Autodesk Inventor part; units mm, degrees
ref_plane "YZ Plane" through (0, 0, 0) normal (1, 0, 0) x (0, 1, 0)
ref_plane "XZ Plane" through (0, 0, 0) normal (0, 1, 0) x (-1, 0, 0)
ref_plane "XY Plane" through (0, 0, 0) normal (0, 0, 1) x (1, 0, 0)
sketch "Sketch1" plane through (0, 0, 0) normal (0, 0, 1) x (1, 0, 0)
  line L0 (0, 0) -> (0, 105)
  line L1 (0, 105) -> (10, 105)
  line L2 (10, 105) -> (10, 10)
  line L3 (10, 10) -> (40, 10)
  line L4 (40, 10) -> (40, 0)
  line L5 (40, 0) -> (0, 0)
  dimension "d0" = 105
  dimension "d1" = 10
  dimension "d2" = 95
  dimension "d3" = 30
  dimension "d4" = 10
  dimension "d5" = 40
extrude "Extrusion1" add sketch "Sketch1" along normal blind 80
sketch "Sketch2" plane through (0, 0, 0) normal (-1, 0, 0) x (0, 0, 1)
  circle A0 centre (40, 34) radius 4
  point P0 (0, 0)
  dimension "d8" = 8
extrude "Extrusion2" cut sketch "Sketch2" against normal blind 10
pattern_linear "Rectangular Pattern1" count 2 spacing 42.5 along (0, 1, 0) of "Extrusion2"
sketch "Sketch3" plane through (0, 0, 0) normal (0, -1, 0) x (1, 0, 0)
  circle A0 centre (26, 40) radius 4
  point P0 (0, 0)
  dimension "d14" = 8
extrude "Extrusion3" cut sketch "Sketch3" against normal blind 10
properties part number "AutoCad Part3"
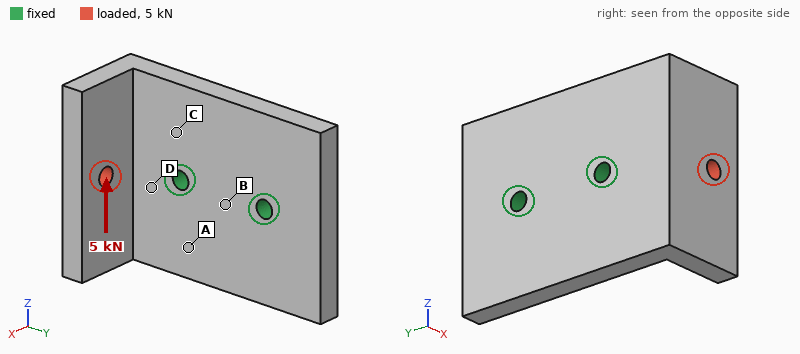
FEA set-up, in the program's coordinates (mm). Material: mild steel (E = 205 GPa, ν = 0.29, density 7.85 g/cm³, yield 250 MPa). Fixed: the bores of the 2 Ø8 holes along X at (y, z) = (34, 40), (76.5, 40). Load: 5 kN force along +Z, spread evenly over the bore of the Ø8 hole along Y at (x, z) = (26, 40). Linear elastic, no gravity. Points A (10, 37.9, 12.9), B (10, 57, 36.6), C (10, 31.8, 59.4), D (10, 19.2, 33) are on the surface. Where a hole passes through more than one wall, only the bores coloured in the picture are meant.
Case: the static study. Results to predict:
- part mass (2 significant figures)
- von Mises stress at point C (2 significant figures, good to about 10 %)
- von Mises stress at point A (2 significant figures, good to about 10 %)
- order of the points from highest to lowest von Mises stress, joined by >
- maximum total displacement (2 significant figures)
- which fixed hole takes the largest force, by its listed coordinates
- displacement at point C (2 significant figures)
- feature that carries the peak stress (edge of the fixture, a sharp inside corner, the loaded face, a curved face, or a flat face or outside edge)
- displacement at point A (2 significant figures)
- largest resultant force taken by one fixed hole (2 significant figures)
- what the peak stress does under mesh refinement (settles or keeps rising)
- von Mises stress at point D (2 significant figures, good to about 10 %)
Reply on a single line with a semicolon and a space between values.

840 g; 42 MPa; 32 MPa; D > C > A > B; 88 µm; (34, 40); 15 µm; edge of the fixture; 19 µm; 7.8 kN; keeps rising; 66 MPa
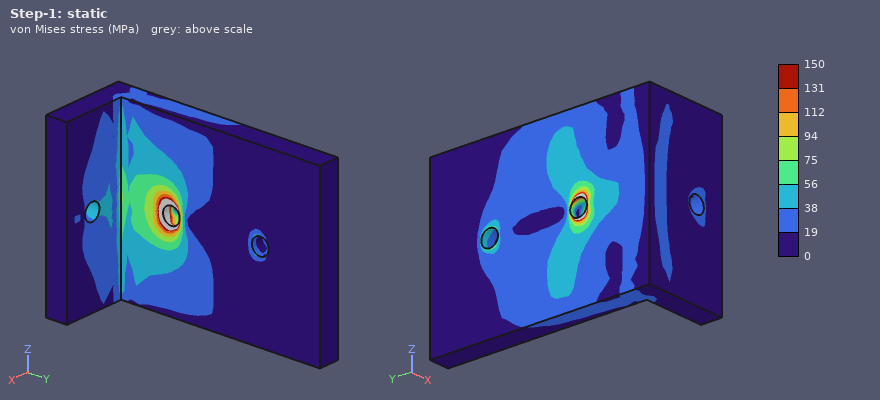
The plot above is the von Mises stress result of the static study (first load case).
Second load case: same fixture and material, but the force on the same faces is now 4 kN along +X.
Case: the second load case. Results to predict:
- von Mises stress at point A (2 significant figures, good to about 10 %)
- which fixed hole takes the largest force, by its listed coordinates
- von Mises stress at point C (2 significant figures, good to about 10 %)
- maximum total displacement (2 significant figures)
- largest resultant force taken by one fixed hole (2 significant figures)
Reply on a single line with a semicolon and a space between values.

35 MPa; (34, 40); 45 MPa; 73 µm; 5.1 kN
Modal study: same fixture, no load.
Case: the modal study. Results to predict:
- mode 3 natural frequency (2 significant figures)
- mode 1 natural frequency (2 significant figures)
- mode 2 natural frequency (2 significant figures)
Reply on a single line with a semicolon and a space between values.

4400 Hz; 2400 Hz; 2400 Hz
